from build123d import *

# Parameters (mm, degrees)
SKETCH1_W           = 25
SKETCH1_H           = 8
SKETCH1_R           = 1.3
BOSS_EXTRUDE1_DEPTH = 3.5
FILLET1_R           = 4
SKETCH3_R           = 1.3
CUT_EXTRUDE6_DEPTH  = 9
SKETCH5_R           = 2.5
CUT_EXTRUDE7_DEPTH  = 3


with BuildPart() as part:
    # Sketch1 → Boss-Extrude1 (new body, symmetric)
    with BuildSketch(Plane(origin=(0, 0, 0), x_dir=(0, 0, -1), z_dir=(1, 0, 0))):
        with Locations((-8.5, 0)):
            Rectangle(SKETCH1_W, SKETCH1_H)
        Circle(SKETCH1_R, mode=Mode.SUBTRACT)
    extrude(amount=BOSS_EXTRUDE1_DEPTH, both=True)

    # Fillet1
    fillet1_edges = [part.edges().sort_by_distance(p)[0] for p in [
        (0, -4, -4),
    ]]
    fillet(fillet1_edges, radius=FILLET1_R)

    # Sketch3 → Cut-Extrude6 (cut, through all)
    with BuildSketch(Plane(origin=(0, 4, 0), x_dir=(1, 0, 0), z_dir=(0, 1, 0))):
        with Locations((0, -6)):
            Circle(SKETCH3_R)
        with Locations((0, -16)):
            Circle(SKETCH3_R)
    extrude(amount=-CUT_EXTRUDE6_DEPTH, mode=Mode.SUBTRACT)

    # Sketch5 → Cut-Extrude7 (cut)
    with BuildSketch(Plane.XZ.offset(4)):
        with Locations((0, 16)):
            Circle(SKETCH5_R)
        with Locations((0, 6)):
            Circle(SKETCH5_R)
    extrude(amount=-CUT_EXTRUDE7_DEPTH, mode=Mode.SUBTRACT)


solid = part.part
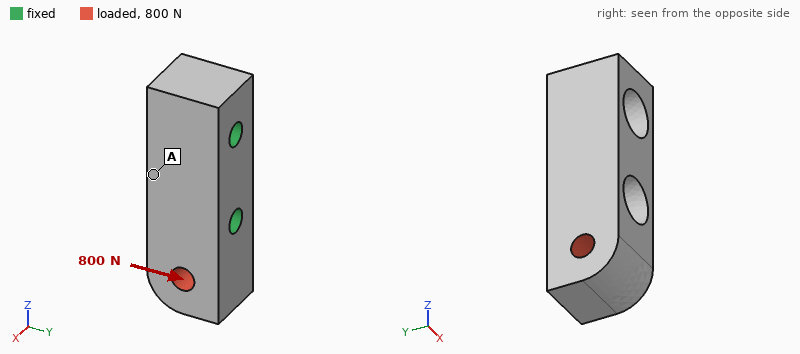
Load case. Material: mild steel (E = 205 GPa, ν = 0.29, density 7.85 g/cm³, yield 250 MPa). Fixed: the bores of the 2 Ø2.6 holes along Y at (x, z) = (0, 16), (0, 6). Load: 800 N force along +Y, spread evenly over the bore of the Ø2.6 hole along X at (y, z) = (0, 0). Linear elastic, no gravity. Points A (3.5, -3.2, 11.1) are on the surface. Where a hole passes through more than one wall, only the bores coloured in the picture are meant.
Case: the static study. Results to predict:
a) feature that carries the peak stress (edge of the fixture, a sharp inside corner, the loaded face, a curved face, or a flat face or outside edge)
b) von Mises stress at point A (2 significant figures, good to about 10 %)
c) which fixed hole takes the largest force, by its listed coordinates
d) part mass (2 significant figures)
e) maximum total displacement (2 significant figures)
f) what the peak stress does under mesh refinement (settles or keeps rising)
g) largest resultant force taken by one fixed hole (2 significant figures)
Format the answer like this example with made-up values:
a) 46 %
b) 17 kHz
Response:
a) edge of the fixture
b) 18 MPa
c) (0, 6)
d) 9.2 g
e) 6.2 µm
f) keeps rising
g) 950 N
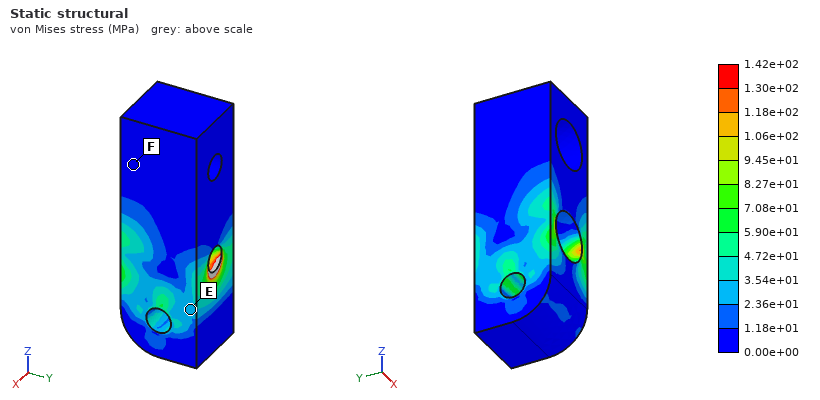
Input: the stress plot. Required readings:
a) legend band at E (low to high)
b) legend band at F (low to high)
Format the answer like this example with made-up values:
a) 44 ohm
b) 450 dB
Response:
a) 2.36e+01 to 3.54e+01 MPa
b) 0.00e+00 to 1.18e+01 MPa
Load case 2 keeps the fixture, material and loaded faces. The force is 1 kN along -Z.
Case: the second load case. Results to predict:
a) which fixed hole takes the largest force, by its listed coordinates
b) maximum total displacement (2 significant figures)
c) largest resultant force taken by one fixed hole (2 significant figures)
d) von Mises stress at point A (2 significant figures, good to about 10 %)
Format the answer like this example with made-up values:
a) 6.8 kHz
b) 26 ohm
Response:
a) (0, 6)
b) 1.9 µm
c) 860 N
d) 9.6 MPa
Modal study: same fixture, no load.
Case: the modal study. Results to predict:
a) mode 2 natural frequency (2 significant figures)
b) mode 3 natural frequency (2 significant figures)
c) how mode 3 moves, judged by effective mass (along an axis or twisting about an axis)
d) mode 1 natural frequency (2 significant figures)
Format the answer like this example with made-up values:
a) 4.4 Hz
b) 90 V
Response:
a) 38 kHz
b) 59 kHz
c) twisting about Z
d) 37 kHz
